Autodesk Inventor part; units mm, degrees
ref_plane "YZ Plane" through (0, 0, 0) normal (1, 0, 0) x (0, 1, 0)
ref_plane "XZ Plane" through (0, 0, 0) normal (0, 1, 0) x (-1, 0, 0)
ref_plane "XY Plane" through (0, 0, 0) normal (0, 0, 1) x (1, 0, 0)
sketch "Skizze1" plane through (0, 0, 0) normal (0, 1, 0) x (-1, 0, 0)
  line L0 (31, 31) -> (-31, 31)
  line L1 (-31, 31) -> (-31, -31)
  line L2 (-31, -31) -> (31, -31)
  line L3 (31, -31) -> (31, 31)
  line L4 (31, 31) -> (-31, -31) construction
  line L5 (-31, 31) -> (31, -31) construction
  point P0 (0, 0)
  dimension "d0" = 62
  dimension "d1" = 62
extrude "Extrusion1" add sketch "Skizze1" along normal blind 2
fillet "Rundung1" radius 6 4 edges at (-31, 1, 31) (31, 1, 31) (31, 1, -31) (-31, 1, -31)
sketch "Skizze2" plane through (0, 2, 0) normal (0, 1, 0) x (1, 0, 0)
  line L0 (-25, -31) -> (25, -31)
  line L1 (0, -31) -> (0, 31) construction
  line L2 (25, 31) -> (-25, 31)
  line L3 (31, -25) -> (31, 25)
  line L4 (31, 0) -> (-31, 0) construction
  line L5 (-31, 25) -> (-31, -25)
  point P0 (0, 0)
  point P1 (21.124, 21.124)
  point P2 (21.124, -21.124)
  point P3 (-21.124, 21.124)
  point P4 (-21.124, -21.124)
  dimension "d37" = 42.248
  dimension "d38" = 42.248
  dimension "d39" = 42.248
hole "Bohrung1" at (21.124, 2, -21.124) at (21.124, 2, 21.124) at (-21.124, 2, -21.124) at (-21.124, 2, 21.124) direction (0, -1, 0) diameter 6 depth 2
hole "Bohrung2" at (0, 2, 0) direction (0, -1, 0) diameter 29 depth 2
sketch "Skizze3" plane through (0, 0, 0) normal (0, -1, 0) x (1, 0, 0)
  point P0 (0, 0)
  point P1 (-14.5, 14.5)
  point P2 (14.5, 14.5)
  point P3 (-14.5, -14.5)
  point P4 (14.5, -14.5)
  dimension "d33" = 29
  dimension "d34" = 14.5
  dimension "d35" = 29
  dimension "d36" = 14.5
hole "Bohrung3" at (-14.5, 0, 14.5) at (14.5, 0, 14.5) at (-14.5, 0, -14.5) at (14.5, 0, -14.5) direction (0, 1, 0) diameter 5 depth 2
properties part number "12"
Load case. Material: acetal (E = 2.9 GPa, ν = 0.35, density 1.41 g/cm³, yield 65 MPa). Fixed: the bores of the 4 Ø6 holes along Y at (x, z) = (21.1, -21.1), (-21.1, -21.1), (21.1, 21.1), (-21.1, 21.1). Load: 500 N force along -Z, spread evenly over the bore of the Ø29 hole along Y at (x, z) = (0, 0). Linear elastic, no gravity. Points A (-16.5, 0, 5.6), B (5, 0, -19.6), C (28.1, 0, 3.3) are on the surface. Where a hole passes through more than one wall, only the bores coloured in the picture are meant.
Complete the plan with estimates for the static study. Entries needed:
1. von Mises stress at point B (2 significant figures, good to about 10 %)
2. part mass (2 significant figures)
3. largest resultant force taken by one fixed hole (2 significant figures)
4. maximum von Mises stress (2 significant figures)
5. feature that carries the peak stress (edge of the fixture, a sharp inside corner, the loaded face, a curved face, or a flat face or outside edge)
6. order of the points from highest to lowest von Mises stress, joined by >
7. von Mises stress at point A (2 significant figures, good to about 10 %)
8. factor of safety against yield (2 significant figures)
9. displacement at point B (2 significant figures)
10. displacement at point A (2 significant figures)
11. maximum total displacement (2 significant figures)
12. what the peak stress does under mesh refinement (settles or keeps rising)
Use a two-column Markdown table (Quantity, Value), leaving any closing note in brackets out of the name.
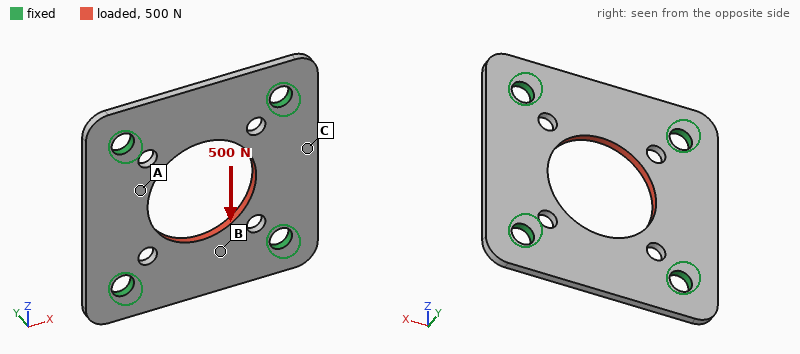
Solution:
| Quantity | Value |
|---|---|
| von Mises stress at point B | 2.3 MPa |
| part mass | 8.3 g |
| largest resultant force taken by one fixed hole | 130 N |
| maximum von Mises stress | 12 MPa |
| feature that carries the peak stress | a curved face |
| order of the points from highest to lowest von Mises stress, joined by > | A > B > C |
| von Mises stress at point A | 4.8 MPa |
| factor of safety against yield | 5.5 |
| displacement at point B | 40 µm |
| displacement at point A | 21 µm |
| maximum total displacement | 47 µm |
| what the peak stress does under mesh refinement | settles |
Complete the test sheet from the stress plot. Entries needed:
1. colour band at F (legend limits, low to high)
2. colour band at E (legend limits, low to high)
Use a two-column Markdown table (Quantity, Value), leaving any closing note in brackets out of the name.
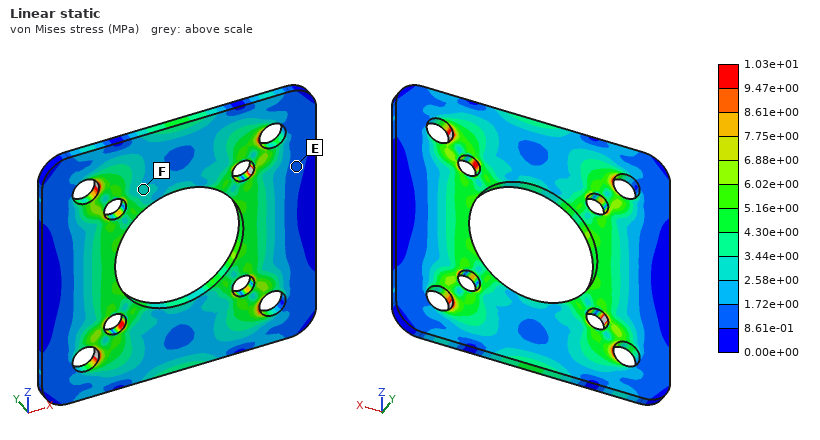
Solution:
| Quantity | Value |
|---|---|
| colour band at F | 2.58e+00 to 3.44e+00 MPa |
| colour band at E | 8.61e-01 to 1.72e+00 MPa |
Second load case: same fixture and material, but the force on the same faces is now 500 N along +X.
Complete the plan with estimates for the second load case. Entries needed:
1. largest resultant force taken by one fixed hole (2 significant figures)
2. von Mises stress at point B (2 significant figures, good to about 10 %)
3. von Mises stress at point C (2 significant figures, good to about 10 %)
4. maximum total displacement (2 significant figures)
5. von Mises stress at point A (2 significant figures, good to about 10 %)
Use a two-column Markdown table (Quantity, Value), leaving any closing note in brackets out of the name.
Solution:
| Quantity | Value |
|---|---|
| largest resultant force taken by one fixed hole | 130 N |
| von Mises stress at point B | 3.5 MPa |
| von Mises stress at point C | 2.6 MPa |
| maximum total displacement | 47 µm |
| von Mises stress at point A | 2.7 MPa |
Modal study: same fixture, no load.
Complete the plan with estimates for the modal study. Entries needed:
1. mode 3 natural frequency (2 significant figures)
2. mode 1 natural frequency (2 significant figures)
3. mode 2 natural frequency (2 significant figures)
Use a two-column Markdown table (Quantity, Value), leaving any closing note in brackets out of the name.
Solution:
| Quantity | Value |
|---|---|
| mode 3 natural frequency | 2000 Hz |
| mode 1 natural frequency | 1900 Hz |
| mode 2 natural frequency | 1900 Hz |
